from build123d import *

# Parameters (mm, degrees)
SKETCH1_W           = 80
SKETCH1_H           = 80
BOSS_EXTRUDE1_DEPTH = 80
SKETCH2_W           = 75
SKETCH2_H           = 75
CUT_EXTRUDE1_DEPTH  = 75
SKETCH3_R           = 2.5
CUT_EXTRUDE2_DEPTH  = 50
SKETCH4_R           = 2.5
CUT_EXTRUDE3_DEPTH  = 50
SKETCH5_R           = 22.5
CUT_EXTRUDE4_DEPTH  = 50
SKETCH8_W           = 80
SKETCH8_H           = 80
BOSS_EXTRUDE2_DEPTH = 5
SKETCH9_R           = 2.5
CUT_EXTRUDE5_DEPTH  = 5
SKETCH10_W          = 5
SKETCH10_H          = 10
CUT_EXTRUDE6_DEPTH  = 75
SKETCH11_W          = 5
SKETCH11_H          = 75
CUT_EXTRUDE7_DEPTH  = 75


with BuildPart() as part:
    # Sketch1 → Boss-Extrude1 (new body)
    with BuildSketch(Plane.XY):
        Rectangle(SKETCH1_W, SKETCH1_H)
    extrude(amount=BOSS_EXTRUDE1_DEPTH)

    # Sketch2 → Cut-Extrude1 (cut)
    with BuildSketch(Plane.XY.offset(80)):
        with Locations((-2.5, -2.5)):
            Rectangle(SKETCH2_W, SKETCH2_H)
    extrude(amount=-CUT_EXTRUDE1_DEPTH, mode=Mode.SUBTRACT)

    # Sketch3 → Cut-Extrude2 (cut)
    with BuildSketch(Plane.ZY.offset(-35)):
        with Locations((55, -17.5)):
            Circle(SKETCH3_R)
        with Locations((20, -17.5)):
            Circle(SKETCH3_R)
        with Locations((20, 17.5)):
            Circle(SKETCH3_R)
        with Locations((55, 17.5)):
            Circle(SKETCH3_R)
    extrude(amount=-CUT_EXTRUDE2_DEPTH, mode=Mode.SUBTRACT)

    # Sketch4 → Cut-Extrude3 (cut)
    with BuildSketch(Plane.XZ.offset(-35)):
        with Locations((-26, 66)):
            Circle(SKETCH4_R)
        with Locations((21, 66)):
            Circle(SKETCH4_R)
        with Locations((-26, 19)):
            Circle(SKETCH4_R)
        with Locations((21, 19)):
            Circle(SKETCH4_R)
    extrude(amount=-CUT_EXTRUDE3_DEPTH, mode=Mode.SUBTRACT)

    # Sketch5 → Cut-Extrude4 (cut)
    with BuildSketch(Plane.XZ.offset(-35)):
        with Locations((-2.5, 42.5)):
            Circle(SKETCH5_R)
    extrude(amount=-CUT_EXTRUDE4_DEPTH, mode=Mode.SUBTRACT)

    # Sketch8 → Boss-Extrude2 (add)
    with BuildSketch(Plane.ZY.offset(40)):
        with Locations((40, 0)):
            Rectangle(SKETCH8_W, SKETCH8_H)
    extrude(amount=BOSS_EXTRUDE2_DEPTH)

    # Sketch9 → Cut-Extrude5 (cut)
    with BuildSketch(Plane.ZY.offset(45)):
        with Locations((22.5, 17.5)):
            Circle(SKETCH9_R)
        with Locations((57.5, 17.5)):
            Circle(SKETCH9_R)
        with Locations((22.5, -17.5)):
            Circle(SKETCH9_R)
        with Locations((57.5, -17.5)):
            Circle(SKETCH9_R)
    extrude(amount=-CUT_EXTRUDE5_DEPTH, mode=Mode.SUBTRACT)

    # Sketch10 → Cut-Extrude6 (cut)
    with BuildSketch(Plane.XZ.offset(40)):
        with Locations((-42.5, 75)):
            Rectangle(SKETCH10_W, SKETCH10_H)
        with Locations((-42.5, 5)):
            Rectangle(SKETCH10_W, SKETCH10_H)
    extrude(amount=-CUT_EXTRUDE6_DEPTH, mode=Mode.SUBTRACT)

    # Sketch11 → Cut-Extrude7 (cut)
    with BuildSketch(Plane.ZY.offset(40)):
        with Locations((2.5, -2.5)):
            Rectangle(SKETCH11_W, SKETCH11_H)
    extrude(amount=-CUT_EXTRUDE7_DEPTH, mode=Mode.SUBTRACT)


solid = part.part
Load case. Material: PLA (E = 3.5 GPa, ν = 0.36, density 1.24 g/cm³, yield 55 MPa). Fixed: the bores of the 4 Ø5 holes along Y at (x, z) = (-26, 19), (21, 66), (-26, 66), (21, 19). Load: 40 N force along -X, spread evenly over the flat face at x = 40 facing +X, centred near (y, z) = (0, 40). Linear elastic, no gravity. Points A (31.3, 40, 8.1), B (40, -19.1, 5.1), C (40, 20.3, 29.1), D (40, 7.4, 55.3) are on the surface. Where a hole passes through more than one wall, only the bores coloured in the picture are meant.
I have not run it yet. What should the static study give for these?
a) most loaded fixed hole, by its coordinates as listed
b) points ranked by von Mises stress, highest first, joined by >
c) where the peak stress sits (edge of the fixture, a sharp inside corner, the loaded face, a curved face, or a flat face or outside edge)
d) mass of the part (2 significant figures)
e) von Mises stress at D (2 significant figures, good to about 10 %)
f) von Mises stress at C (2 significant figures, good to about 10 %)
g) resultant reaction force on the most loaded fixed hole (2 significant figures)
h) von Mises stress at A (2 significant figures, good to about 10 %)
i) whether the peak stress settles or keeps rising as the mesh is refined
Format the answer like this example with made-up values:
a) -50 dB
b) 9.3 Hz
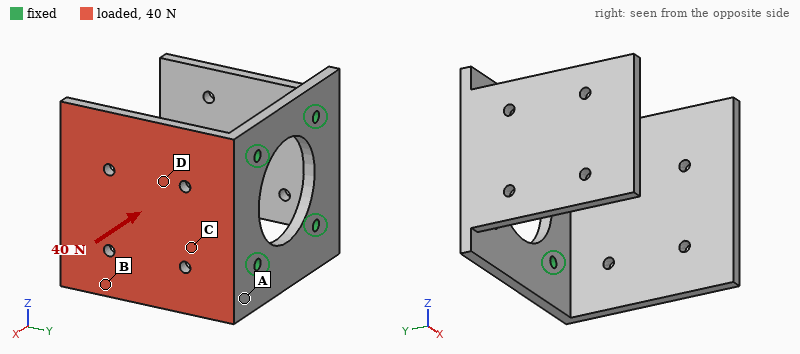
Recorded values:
a) (21, 19)
b) A > C > D > B
c) edge of the fixture
d) 96 g
e) 1.4 MPa
f) 2.6 MPa
g) 24 N
h) 3.9 MPa
i) keeps rising
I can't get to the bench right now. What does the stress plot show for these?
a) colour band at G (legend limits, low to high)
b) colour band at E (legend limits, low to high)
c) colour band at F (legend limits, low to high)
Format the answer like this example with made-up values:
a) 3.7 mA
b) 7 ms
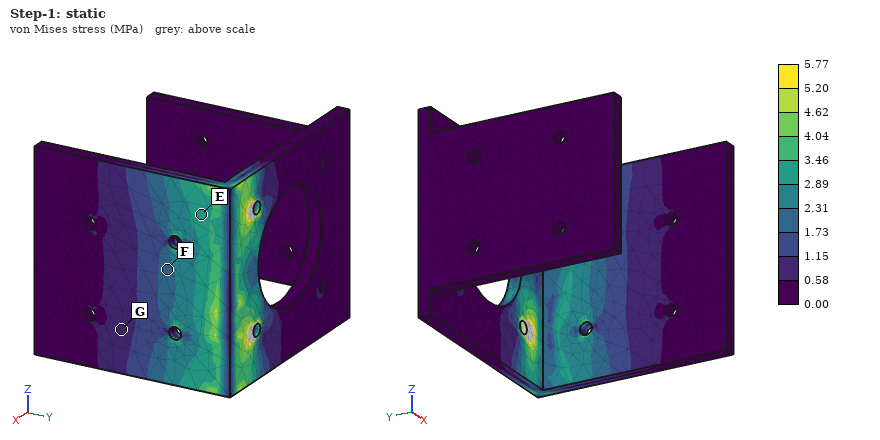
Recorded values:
a) 0.58 to 1.15 MPa
b) 2.89 to 3.46 MPa
c) 1.73 to 2.31 MPa
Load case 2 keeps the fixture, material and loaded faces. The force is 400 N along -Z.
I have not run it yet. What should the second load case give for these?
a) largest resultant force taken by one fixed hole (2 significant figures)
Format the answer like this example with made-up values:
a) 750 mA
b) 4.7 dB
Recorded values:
a) 380 N
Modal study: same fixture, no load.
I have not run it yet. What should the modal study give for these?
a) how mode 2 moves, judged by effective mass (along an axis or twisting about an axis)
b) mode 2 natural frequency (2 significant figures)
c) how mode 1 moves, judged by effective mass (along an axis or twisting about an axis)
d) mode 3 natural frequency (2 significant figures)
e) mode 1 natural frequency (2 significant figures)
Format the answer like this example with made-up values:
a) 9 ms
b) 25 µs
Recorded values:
a) along X
b) 180 Hz
c) along X
d) 450 Hz
e) 170 Hz
